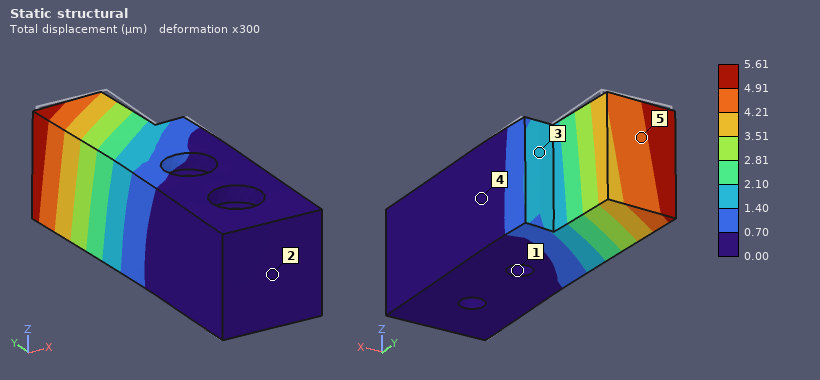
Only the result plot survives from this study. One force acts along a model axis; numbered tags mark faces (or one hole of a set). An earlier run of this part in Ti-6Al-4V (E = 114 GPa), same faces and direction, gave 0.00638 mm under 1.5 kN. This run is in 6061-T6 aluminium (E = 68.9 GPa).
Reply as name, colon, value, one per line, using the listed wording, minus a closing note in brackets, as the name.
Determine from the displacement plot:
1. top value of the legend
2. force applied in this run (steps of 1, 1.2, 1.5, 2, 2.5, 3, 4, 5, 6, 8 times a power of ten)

top value of the legend: 5.61 µm
force applied in this run: 800 N
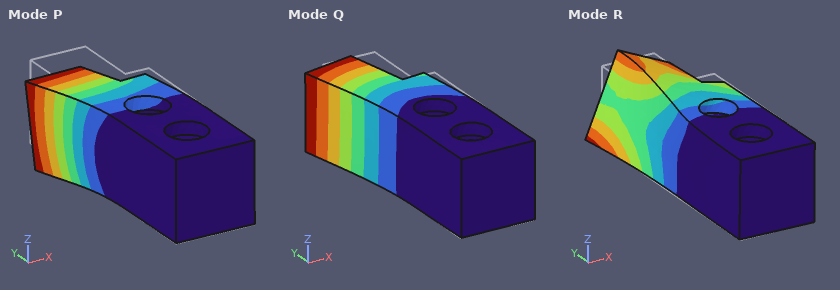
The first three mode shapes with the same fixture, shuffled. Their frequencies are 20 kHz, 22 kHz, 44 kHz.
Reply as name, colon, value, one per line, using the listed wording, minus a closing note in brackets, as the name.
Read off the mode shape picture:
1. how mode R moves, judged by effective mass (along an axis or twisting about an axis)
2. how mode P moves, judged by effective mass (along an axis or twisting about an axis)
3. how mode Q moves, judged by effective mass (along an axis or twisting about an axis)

how mode R moves, judged by effective mass: twisting about Y
how mode P moves, judged by effective mass: along Z
how mode Q moves, judged by effective mass: along X
